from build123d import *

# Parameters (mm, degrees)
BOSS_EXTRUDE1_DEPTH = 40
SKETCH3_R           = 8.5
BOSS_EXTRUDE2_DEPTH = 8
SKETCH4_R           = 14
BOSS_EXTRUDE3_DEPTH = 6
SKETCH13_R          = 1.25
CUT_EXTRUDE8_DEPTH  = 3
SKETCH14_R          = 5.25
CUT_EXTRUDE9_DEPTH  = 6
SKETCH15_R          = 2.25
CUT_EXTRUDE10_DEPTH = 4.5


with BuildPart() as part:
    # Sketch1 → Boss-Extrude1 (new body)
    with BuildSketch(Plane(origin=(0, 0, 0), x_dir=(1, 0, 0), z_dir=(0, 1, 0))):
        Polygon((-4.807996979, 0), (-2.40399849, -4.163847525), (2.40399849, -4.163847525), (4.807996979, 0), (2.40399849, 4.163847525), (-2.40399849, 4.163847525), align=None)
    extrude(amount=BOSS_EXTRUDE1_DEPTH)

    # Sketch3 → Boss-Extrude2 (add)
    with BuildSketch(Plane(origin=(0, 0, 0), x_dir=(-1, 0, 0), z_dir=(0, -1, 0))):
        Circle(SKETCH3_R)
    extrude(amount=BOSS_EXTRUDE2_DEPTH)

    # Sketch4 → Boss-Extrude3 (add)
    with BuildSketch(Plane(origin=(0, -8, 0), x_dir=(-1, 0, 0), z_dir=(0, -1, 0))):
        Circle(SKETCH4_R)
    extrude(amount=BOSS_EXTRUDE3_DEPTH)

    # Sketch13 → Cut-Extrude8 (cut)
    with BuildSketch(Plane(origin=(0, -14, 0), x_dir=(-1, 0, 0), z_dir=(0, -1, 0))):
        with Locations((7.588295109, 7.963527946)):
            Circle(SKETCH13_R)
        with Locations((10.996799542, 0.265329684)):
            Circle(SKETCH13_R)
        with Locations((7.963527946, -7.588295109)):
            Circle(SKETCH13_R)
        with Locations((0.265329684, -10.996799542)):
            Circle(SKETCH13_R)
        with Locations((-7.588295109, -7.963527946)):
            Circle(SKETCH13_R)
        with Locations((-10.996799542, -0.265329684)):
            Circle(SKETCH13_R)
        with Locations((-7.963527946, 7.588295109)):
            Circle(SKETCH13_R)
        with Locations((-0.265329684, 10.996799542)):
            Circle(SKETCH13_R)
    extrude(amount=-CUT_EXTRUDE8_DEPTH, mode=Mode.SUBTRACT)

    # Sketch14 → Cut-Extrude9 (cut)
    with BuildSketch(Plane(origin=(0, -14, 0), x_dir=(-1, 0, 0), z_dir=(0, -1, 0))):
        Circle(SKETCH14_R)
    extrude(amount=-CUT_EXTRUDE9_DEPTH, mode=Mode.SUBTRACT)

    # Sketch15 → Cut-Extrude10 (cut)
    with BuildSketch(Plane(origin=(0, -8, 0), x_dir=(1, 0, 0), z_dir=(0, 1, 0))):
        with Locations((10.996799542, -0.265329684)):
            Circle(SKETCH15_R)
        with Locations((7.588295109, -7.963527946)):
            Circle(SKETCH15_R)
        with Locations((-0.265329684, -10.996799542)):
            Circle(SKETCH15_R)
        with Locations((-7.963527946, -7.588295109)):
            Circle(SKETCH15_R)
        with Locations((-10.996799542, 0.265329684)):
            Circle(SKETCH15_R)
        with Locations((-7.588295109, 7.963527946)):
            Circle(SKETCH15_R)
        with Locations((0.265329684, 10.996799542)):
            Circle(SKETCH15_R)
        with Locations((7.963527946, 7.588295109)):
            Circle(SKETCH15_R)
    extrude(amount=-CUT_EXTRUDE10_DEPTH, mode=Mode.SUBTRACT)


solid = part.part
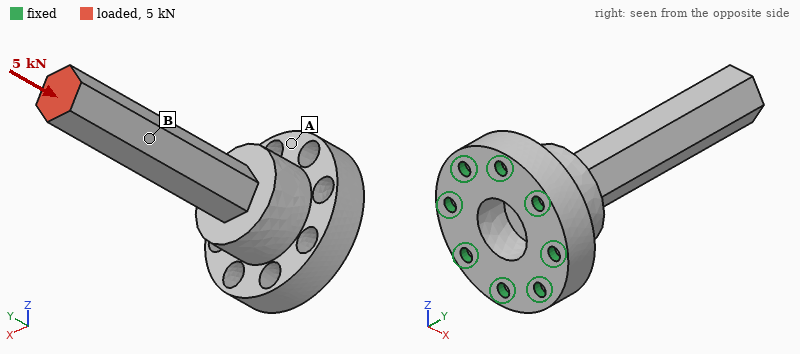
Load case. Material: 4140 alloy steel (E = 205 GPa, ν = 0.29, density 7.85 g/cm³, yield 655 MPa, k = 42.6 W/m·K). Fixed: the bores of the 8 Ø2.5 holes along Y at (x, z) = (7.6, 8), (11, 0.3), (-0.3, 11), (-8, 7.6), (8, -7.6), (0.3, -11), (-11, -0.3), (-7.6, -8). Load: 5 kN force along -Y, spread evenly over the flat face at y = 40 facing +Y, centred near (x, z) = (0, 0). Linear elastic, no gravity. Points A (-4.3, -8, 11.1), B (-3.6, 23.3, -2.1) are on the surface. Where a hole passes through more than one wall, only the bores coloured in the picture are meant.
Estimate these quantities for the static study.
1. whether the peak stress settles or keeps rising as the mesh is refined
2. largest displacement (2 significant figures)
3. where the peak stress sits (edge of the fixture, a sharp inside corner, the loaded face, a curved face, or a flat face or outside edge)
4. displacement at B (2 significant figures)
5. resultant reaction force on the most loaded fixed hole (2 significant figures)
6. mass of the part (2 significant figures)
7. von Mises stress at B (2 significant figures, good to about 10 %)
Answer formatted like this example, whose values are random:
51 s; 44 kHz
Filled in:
keeps rising; 20 µm; edge of the fixture; 14 µm; 730 N; 53 g; 83 MPa
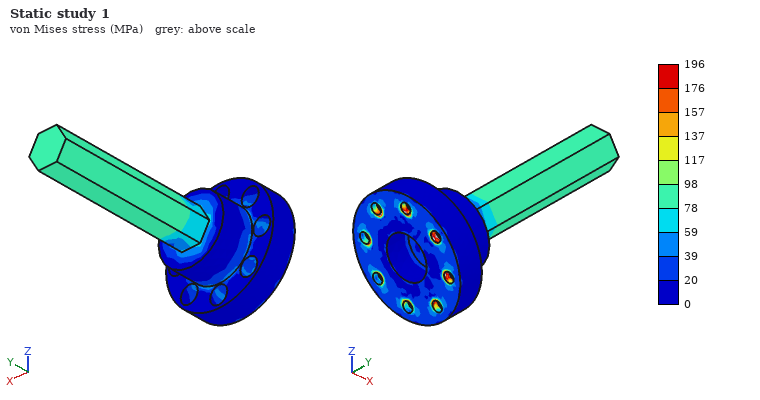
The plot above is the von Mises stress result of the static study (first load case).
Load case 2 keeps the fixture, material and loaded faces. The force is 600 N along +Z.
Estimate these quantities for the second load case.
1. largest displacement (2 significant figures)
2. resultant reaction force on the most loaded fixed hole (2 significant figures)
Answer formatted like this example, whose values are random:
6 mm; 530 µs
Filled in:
0.28 mm; 790 N
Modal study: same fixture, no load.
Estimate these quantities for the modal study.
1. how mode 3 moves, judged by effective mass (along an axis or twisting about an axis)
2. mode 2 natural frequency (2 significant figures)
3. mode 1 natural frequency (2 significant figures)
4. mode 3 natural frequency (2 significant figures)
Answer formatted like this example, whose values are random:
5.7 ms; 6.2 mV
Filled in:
along Z; 3300 Hz; 3300 Hz; 17 kHz
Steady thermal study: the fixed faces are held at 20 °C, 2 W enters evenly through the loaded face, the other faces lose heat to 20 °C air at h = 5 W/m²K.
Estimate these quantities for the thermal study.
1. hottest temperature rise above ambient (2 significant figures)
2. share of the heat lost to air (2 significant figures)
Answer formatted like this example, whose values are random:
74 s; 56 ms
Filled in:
35 K; 6.3 %
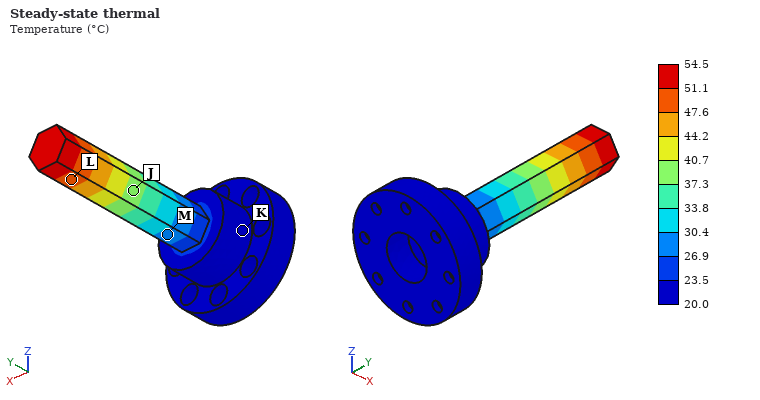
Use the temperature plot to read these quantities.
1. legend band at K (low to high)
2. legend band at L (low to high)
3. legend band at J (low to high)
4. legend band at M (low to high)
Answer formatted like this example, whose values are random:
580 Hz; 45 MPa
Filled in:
20.0 to 23.5 °C; 47.6 to 51.1 °C; 37.3 to 40.7 °C; 26.9 to 30.4 °C
